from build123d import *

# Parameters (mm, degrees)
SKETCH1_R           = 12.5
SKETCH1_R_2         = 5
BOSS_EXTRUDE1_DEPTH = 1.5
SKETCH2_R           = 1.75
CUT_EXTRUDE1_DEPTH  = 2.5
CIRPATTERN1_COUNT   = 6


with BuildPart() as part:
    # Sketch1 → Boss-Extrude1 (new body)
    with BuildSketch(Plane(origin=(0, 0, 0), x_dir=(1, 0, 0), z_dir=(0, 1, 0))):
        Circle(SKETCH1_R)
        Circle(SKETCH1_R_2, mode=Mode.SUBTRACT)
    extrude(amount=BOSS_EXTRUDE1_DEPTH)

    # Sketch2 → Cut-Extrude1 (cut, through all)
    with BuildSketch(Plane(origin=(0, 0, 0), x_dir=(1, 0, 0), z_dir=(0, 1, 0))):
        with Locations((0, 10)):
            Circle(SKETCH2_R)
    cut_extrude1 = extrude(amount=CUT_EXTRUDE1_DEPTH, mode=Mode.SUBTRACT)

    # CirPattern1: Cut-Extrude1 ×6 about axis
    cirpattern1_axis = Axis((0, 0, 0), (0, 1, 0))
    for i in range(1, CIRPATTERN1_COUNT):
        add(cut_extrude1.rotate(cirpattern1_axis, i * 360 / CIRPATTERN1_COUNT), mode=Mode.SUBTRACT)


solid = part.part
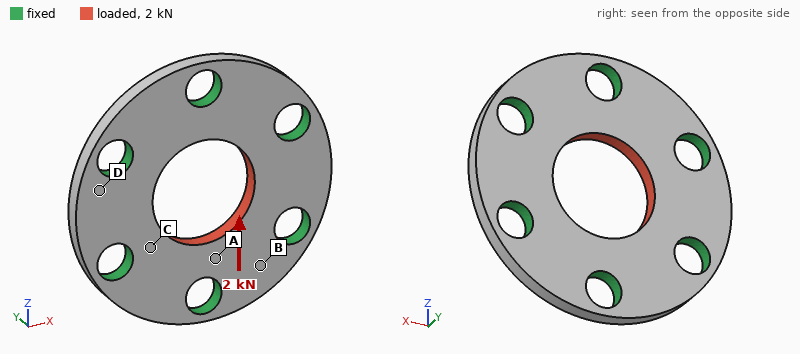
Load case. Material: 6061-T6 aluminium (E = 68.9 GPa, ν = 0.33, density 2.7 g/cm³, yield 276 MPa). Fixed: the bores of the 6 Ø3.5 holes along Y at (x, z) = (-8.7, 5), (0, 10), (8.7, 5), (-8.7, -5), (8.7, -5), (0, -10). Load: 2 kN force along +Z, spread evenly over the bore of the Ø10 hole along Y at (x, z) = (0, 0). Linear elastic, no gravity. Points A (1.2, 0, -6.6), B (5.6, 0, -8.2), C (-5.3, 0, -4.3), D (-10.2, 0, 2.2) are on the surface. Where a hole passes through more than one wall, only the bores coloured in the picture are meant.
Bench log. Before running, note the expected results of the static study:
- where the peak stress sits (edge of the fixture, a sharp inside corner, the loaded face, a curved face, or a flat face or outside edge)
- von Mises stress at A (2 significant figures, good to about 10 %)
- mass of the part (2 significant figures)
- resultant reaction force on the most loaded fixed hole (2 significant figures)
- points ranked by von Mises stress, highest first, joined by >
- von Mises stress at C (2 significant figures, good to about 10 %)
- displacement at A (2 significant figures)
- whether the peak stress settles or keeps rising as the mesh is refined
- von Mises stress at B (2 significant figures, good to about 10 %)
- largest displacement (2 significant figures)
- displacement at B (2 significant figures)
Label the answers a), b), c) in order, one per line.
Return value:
a) edge of the fixture
b) 52 MPa
c) 1.4 g
d) 480 N
e) A > C > B > D
f) 31 MPa
g) 1.6 µm
h) keeps rising
i) 12 MPa
j) 3.5 µm
k) 1.4 µm
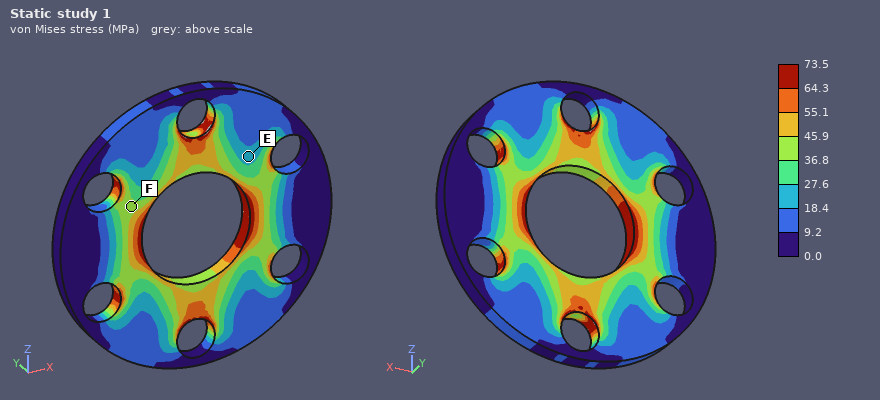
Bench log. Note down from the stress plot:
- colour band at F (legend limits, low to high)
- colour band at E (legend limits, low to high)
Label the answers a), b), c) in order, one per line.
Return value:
a) 36.8 to 45.9 MPa
b) 18.4 to 27.6 MPa
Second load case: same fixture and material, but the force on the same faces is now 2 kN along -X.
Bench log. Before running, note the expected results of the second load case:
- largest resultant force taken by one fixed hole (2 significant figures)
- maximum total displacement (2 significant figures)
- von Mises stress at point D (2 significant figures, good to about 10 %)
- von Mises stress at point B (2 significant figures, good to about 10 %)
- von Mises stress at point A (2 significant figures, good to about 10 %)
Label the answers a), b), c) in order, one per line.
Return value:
a) 430 N
b) 3.7 µm
c) 23 MPa
d) 7.5 MPa
e) 31 MPa
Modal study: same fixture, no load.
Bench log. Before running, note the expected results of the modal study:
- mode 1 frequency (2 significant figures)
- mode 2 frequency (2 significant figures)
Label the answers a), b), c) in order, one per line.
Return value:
a) 81 kHz
b) 89 kHz
